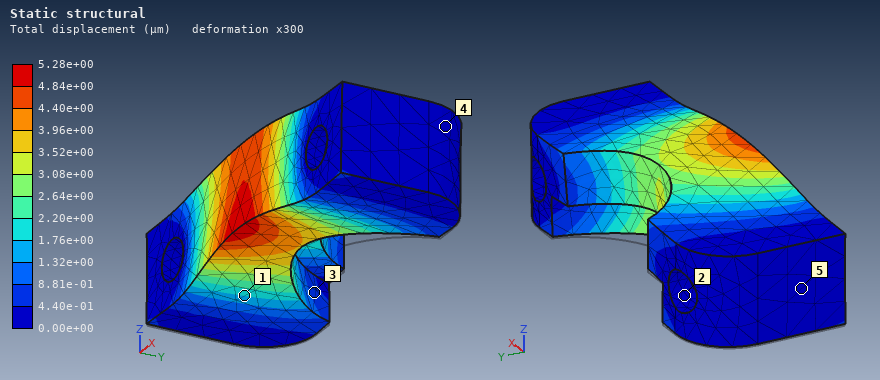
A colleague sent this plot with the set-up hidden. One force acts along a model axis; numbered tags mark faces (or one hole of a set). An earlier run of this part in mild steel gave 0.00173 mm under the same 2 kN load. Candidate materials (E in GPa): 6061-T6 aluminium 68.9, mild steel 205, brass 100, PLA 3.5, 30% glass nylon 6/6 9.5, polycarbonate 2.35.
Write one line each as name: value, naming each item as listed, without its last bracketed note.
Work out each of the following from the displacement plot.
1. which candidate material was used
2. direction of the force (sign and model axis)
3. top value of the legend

which candidate material was used: 6061-T6 aluminium
direction of the force: +Z
top value of the legend: 5.28e+00 µm
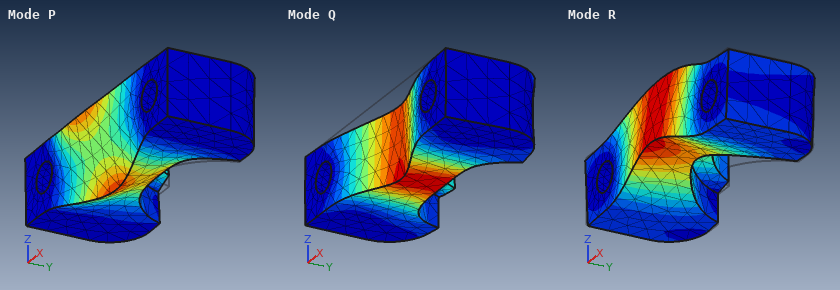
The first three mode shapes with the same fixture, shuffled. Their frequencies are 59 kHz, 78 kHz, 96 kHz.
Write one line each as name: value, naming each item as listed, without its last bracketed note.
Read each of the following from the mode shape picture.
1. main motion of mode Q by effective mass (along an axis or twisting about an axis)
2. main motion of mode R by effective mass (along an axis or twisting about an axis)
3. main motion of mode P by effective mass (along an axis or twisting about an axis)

main motion of mode Q by effective mass: along Y
main motion of mode R by effective mass: along Z
main motion of mode P by effective mass: twisting about X
